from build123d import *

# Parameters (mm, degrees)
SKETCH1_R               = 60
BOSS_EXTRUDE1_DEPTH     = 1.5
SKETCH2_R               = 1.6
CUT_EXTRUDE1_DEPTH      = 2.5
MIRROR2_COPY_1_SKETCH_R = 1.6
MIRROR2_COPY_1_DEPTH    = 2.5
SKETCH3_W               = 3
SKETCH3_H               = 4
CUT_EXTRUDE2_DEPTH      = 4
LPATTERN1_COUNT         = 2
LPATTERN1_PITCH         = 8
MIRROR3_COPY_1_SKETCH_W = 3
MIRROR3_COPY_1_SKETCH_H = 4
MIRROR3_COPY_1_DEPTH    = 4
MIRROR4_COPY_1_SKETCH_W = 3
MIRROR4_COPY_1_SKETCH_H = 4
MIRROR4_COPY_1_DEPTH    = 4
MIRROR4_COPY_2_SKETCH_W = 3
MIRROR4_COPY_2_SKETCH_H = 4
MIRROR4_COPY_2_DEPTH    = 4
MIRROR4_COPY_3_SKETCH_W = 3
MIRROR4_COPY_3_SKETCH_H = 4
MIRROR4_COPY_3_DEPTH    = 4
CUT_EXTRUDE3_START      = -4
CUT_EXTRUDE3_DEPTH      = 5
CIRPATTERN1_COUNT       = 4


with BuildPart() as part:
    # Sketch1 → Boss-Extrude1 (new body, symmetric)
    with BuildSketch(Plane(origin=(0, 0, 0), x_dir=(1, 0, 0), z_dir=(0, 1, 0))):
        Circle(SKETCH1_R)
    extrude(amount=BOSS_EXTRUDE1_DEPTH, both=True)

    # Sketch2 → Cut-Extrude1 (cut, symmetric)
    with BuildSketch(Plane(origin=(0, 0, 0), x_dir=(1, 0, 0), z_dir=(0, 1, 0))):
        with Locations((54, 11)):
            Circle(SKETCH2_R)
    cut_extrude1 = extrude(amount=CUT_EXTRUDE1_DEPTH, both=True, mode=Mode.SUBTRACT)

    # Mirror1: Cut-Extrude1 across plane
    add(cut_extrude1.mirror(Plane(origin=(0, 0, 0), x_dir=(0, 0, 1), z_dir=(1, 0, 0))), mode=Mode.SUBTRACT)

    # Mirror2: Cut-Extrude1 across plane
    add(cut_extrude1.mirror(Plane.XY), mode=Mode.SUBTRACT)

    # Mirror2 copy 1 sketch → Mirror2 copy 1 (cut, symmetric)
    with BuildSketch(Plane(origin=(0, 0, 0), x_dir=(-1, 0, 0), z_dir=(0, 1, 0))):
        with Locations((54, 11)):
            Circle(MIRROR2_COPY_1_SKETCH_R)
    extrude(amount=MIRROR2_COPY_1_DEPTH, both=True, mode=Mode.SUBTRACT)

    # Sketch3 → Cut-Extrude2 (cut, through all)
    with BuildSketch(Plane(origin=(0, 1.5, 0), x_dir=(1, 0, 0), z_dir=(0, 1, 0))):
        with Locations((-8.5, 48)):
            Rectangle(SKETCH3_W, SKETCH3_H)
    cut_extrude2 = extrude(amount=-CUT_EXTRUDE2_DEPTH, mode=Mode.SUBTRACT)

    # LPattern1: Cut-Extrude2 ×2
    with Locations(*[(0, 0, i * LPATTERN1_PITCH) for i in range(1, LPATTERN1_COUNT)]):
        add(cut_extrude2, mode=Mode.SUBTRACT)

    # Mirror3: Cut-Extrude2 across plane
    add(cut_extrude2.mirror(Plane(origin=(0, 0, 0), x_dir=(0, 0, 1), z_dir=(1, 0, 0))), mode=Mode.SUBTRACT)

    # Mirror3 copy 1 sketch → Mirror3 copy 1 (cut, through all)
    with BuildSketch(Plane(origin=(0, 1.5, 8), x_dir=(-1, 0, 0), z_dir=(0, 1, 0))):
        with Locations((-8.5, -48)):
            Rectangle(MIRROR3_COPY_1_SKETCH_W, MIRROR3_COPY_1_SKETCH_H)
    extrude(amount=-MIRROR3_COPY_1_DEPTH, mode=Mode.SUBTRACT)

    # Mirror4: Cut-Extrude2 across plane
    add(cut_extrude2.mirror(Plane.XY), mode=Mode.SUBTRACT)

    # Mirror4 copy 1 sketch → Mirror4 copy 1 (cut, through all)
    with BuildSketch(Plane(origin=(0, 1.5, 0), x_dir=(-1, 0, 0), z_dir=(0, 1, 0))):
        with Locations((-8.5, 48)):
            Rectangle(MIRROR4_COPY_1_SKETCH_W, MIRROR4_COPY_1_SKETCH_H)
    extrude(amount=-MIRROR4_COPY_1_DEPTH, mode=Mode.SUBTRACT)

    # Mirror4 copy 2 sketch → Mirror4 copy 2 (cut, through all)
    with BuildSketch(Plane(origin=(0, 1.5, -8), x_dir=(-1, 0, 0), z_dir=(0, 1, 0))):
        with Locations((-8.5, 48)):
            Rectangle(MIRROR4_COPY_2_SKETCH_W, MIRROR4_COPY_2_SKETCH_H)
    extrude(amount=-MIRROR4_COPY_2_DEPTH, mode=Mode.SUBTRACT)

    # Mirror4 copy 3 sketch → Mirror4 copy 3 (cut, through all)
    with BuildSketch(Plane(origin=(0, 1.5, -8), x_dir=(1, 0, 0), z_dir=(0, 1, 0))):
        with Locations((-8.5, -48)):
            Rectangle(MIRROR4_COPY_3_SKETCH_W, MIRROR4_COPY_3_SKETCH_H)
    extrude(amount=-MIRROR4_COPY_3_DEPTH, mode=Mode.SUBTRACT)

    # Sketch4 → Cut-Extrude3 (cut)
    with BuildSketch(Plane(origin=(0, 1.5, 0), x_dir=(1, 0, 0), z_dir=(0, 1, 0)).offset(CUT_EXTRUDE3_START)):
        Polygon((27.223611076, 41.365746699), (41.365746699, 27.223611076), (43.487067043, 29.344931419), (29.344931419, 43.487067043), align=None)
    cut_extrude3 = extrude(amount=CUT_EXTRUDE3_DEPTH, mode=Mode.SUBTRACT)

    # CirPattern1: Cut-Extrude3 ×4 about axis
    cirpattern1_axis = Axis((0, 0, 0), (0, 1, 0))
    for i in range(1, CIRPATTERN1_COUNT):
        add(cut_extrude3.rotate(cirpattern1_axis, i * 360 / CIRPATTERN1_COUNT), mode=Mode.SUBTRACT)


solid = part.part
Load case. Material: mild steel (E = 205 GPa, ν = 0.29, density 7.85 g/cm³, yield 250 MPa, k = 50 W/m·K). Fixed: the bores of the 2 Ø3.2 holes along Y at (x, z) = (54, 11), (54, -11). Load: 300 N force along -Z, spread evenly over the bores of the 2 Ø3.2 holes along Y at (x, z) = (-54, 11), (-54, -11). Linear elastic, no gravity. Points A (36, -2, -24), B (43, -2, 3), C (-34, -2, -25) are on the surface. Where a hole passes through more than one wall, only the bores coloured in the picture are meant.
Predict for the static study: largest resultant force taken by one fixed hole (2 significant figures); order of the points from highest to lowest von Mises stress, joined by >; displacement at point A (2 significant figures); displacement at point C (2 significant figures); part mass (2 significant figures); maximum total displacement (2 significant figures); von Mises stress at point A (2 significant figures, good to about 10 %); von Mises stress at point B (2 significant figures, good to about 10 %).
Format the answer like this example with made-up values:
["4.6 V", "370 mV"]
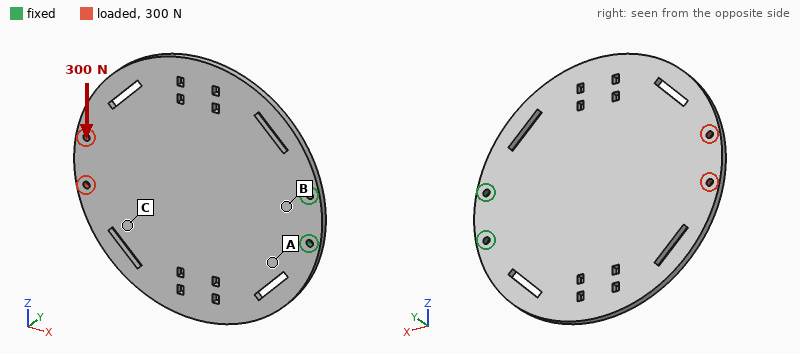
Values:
["1.3 kN", "B > A > C", "7.5 µm", "26 µm", "260 g", "32 µm", "8.0 MPa", "21 MPa"]
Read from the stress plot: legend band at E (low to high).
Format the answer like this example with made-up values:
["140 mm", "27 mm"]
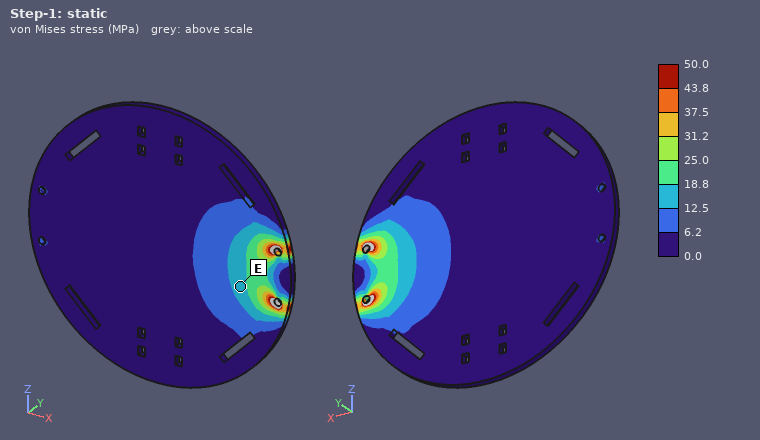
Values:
["12.5 to 18.8 MPa"]
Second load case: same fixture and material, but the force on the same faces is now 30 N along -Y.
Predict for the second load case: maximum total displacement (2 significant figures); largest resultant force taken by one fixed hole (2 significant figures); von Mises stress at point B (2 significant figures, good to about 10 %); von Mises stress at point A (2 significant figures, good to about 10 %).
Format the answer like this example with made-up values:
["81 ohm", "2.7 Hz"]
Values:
["0.41 mm", "15 N", "29 MPa", "23 MPa"]
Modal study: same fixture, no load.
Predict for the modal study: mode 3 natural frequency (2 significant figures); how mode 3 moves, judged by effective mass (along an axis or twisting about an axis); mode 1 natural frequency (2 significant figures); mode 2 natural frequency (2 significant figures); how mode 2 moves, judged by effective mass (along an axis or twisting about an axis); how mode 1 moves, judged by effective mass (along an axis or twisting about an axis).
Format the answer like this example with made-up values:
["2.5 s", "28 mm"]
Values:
["930 Hz", "along Y", "180 Hz", "390 Hz", "twisting about X", "along Y"]
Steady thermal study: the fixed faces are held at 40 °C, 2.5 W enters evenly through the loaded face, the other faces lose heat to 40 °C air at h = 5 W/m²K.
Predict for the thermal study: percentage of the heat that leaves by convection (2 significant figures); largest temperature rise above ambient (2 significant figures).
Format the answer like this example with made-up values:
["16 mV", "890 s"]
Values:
["41 %", "21 K"]
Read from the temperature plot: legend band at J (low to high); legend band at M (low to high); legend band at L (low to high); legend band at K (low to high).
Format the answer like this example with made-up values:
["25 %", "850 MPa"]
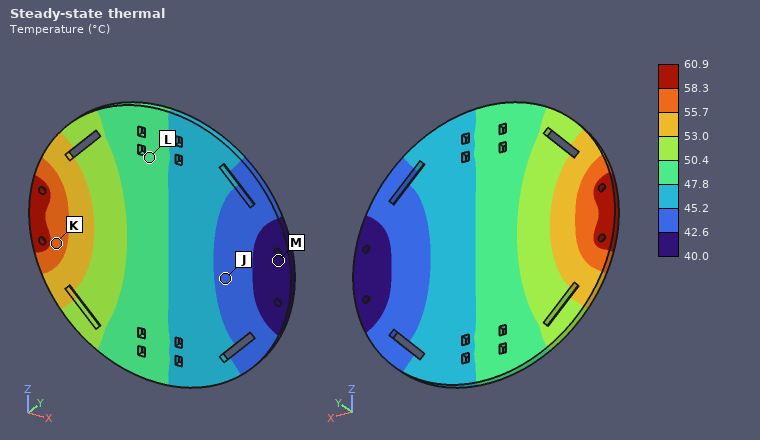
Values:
["42.6 to 45.2 °C", "40.0 to 42.6 °C", "47.8 to 50.4 °C", "55.7 to 58.3 °C"]
